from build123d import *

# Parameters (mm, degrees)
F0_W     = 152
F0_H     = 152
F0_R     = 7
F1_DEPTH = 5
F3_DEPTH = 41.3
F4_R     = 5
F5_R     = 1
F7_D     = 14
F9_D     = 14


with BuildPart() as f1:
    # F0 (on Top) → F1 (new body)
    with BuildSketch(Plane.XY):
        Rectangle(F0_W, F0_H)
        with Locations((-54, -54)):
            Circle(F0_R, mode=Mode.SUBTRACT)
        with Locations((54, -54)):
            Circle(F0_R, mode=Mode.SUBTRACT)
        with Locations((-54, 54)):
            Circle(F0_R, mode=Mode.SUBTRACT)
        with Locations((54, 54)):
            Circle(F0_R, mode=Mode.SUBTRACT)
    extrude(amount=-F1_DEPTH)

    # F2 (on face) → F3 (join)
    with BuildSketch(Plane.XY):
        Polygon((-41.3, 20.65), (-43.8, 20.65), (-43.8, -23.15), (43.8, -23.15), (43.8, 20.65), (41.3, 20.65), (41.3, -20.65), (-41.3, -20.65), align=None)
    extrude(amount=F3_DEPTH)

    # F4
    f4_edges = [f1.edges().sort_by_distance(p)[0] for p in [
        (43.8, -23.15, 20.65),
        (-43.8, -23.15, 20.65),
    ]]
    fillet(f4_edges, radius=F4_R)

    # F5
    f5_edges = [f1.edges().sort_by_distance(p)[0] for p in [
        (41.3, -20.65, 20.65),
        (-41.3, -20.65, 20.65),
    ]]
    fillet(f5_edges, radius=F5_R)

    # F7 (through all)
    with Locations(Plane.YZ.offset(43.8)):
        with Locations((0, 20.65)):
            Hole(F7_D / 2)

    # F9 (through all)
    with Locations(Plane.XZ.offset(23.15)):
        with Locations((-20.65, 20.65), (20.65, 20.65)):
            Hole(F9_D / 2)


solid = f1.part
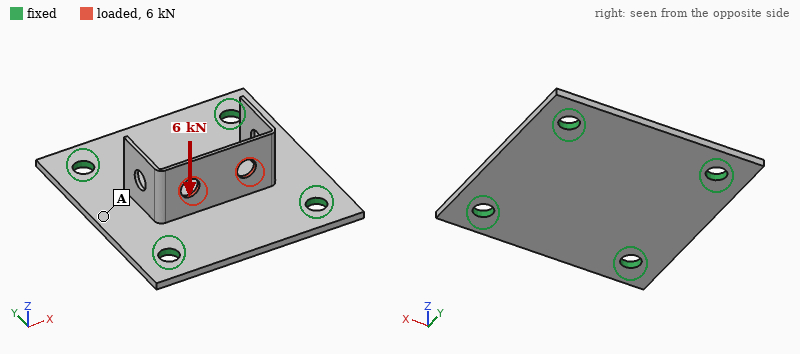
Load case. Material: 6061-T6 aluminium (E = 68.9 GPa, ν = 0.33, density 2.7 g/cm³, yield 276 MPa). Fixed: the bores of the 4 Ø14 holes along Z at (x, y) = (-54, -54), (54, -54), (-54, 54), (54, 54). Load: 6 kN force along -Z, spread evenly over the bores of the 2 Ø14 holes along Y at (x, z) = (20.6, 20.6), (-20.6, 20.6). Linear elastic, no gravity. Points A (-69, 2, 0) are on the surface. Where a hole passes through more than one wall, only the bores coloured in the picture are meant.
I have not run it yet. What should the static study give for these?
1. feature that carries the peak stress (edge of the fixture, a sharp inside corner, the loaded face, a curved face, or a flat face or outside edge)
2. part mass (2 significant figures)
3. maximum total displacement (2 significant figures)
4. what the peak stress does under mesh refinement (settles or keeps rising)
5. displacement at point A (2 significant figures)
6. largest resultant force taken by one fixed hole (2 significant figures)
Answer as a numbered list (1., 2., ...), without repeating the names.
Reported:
1. a sharp inside corner
2. 350 g
3. 0.32 mm
4. keeps rising
5. 0.11 mm
6. 2.4 kN
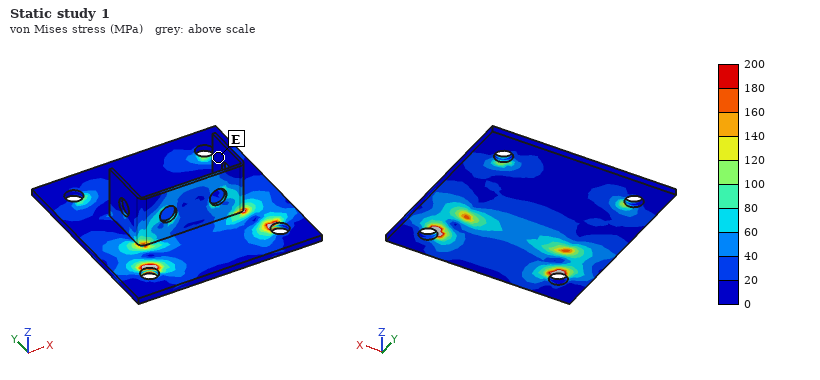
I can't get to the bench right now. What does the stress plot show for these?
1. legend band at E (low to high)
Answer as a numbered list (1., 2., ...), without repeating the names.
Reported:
1. 0 to 20 MPa
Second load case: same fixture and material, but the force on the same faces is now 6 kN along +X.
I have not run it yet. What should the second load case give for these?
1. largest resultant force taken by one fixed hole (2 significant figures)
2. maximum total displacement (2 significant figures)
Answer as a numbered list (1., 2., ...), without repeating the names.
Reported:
1. 2.5 kN
2. 0.22 mm
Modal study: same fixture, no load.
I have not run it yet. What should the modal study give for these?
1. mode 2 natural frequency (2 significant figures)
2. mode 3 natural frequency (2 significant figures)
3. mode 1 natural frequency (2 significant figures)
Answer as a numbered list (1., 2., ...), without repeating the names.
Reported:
1. 1900 Hz
2. 2000 Hz
3. 1700 Hz
